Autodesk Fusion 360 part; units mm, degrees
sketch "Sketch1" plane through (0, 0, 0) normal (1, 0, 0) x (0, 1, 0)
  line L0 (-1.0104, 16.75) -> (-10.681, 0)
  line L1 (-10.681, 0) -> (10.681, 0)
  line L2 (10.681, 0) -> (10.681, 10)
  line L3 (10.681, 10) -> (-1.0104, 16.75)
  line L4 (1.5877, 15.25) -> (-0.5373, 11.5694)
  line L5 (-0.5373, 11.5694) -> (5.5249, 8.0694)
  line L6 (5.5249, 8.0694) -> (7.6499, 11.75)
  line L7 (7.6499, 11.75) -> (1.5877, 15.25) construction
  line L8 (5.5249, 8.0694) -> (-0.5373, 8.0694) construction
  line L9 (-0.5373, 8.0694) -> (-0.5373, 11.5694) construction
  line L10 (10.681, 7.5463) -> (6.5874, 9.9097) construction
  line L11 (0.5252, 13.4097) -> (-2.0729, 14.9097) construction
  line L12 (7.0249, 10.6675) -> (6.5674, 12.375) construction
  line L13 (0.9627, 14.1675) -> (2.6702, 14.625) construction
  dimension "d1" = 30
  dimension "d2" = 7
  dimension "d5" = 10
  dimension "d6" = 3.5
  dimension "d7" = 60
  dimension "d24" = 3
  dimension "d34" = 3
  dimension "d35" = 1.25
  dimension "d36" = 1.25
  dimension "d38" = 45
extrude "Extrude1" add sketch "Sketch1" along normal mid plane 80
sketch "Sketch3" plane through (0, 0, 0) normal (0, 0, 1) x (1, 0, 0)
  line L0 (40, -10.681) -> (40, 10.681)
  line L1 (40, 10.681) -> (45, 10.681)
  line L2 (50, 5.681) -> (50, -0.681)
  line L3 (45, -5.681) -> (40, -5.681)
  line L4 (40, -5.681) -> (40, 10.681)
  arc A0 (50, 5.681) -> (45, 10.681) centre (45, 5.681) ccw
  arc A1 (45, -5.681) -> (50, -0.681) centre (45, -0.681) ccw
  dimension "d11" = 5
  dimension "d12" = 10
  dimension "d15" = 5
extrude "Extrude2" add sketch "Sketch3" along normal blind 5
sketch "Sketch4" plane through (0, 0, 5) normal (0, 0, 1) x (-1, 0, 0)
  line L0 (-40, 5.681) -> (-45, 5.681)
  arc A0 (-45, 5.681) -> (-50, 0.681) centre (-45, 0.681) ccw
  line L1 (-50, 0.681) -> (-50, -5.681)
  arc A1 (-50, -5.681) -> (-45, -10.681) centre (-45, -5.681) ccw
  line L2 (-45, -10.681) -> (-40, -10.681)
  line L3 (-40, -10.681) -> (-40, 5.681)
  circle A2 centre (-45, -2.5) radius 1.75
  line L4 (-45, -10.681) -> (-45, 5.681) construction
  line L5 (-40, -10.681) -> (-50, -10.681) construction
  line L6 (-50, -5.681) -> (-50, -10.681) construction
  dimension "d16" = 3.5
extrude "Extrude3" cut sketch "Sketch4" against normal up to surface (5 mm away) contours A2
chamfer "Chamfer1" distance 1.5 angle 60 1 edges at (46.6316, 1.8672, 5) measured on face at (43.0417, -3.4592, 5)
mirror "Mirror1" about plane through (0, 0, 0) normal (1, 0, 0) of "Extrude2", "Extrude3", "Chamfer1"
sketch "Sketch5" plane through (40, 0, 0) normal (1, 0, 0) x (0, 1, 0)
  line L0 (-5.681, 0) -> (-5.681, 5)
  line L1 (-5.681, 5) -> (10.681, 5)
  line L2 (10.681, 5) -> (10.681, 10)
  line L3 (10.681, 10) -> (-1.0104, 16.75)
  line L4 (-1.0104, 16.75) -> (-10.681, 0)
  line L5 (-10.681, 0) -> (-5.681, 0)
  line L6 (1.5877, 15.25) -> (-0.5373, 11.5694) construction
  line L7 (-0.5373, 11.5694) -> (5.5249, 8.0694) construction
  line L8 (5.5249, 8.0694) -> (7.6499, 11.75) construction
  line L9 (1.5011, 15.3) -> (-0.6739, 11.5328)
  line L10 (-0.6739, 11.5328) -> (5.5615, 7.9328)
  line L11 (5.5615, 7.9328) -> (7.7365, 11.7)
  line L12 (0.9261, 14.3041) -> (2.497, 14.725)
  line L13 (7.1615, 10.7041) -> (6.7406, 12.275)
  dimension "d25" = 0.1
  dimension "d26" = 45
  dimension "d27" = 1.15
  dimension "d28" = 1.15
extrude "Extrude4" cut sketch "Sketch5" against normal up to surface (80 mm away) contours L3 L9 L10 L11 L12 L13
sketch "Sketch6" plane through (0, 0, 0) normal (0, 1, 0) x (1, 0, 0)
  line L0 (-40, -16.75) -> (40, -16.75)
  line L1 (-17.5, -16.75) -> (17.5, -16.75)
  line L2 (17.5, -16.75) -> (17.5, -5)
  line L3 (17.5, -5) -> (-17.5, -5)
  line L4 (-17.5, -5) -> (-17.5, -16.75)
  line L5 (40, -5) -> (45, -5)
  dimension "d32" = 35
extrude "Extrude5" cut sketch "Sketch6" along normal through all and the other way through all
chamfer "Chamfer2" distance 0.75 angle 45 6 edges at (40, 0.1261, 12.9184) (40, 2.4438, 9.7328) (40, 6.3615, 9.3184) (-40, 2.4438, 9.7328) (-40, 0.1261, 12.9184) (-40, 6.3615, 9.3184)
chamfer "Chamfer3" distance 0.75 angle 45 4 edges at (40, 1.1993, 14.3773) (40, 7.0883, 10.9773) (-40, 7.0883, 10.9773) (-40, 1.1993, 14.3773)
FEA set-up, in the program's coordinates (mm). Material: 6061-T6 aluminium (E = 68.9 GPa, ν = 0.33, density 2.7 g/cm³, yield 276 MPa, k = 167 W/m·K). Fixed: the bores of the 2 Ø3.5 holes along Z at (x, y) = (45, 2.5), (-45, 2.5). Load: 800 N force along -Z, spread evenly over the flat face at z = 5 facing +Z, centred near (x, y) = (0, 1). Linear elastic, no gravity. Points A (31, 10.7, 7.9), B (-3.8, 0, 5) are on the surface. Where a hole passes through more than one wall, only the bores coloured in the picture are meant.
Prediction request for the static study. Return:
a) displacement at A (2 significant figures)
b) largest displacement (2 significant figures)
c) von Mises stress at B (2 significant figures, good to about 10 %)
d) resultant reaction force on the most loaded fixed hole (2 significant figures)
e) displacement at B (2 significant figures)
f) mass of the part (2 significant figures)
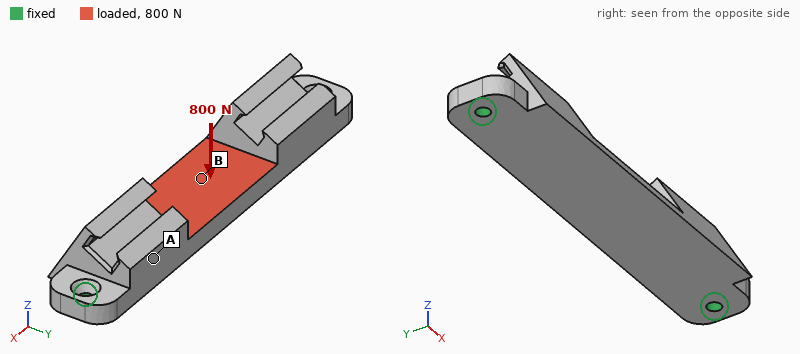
0.097 mm
0.27 mm
88 MPa
750 N
0.26 mm
38 g
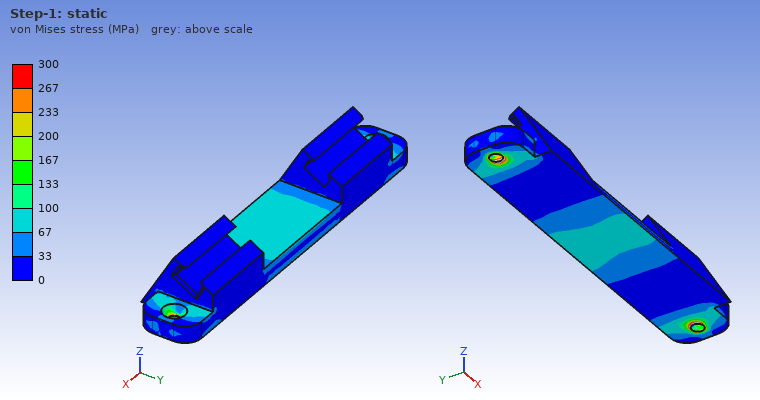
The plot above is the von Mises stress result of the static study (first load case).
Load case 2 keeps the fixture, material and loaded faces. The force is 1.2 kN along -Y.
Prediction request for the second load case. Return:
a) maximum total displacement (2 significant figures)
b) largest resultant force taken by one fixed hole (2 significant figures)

70 µm
680 N
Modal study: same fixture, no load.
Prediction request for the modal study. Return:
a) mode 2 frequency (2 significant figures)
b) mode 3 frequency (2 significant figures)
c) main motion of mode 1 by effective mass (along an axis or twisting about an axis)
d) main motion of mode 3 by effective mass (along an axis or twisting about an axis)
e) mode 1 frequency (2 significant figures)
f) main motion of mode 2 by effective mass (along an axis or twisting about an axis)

4900 Hz
6500 Hz
along Z
along Y
2300 Hz
along Y
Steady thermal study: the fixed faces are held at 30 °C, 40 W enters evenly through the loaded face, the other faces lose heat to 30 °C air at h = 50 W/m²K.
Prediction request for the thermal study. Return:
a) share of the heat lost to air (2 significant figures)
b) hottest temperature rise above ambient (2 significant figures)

14 %
36 K
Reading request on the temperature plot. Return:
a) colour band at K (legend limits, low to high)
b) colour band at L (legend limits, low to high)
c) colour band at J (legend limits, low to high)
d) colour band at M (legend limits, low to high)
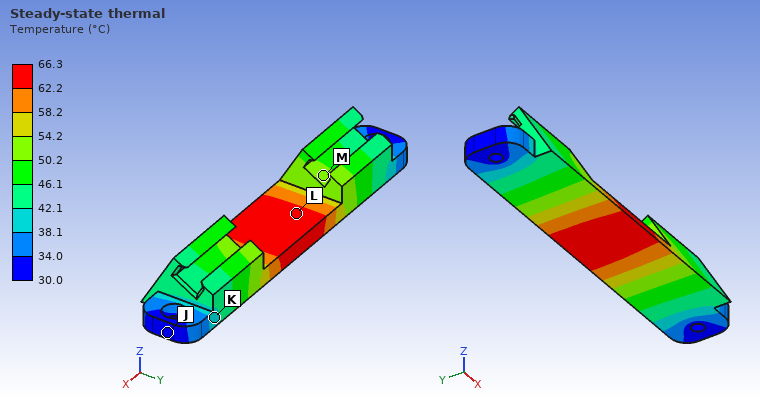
38.1 to 42.1 °C
62.2 to 66.3 °C
30.0 to 34.0 °C
50.2 to 54.2 °C
